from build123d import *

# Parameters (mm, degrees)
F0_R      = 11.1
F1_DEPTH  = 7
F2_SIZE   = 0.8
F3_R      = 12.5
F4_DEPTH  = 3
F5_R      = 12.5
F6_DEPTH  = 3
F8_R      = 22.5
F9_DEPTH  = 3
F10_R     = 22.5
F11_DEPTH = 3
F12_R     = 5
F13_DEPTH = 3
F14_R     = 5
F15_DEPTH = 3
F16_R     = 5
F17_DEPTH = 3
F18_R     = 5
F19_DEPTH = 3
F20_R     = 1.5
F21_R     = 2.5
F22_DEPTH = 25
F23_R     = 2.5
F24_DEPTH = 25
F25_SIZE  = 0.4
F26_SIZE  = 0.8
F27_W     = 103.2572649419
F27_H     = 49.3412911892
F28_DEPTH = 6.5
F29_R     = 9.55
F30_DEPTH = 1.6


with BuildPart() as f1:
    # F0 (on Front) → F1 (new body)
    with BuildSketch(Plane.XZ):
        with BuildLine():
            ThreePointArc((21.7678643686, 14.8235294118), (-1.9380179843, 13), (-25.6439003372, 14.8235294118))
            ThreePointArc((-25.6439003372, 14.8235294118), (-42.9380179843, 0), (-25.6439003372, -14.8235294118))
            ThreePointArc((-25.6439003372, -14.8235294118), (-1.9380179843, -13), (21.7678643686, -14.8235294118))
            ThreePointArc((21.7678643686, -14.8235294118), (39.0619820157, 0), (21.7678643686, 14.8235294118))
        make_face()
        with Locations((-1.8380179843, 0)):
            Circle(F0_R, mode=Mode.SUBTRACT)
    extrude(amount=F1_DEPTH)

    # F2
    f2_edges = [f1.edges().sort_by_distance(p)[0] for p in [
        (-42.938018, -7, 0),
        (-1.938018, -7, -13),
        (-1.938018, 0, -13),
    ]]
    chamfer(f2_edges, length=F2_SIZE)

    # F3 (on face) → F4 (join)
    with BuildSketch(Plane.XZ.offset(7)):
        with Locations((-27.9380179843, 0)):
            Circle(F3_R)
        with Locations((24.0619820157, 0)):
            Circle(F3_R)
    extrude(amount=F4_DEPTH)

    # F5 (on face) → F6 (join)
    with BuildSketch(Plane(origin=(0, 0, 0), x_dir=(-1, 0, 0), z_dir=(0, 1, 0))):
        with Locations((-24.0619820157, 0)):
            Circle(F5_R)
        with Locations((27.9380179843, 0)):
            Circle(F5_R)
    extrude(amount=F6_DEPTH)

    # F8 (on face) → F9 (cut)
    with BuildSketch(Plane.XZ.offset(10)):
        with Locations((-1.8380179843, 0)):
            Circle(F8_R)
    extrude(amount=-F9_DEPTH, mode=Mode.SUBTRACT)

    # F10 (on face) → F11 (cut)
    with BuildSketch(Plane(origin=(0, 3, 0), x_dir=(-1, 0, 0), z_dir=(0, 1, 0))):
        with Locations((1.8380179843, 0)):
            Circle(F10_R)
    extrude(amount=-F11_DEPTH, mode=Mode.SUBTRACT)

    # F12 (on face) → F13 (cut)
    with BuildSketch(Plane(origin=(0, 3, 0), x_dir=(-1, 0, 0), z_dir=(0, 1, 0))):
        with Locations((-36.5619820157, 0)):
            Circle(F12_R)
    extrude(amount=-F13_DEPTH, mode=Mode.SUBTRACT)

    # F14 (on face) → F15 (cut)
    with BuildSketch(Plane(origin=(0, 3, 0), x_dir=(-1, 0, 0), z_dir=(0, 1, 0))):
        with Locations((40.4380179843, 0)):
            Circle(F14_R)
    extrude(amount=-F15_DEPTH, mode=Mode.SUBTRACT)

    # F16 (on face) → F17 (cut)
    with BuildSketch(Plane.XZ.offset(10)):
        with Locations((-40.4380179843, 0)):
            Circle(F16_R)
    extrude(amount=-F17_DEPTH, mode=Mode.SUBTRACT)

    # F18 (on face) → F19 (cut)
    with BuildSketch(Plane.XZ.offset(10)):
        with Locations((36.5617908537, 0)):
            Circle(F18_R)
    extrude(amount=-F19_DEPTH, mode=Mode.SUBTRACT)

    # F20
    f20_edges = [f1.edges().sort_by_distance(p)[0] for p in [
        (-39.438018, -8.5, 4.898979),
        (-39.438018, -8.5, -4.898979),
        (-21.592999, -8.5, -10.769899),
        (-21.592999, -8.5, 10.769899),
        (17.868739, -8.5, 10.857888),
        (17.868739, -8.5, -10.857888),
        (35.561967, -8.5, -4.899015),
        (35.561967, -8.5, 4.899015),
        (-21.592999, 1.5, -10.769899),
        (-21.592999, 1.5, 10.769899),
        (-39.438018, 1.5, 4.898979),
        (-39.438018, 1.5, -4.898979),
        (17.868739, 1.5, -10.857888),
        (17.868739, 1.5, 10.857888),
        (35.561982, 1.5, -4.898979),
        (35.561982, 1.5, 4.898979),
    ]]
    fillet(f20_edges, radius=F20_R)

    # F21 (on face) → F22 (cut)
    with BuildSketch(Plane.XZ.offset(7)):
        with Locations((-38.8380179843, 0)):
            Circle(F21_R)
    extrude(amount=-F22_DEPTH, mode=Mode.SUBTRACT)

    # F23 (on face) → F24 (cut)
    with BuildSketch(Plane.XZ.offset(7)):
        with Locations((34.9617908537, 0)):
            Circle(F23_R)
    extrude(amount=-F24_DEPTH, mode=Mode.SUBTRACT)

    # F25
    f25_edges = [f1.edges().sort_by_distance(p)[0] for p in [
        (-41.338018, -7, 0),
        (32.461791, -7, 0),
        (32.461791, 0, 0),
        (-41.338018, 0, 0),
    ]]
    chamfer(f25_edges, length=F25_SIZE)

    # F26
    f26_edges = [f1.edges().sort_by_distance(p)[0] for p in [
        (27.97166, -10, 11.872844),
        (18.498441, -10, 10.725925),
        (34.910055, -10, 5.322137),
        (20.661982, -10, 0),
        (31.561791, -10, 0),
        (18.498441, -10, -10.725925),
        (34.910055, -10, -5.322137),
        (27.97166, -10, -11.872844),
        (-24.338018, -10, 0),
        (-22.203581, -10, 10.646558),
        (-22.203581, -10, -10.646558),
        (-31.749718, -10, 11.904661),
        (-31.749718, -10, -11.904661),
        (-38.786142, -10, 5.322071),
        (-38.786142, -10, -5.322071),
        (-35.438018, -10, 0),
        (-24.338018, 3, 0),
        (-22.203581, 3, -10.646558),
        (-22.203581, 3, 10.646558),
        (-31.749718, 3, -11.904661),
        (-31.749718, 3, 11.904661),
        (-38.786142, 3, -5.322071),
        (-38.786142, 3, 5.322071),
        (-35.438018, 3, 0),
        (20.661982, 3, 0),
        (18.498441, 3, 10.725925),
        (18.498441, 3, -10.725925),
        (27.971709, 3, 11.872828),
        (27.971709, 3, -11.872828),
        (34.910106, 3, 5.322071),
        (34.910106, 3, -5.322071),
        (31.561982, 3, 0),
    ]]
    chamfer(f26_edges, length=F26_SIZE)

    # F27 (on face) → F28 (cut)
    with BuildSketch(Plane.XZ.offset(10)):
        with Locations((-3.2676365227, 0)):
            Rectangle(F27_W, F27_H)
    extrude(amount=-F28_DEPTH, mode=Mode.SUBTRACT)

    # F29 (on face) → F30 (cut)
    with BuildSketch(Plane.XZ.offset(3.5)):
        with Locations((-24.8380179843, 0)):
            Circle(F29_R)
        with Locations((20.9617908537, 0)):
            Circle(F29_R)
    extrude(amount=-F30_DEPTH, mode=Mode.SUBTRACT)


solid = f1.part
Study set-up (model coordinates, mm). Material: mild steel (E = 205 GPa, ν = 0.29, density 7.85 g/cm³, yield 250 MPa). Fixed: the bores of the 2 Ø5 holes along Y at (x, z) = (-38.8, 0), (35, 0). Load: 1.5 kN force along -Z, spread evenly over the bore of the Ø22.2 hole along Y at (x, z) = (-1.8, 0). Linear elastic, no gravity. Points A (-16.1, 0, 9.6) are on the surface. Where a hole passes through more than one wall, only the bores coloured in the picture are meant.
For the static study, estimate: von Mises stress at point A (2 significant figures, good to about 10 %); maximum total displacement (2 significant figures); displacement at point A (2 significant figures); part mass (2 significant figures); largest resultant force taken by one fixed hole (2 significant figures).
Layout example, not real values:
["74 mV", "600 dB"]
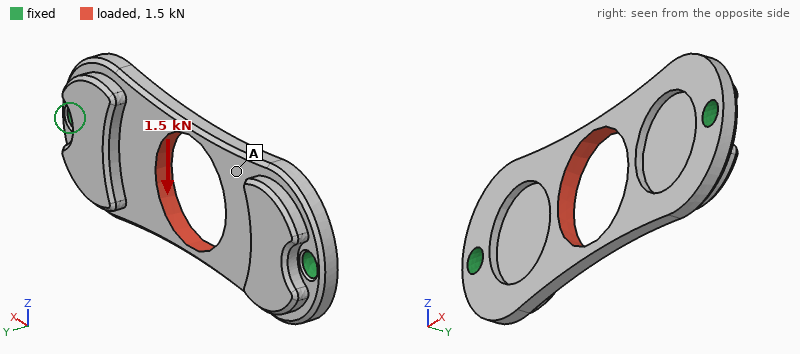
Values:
["19 MPa", "25 µm", "14 µm", "54 g", "750 N"]
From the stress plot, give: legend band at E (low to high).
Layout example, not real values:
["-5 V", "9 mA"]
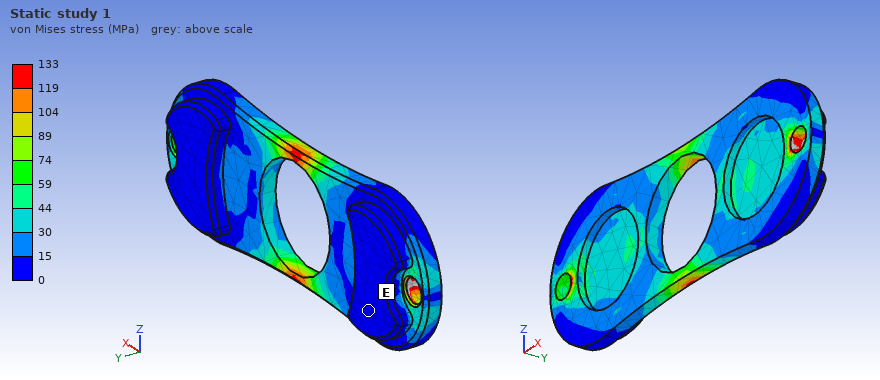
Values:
["0 to 15 MPa"]
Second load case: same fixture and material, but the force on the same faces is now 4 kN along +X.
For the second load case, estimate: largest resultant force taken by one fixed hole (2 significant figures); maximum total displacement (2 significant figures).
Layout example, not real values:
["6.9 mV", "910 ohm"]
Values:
["2.0 kN", "7.3 µm"]
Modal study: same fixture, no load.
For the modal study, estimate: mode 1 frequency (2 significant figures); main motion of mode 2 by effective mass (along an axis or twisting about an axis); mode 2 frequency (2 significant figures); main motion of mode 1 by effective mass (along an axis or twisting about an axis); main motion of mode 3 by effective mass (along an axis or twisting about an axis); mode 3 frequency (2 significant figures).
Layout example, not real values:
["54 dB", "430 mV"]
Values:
["4100 Hz", "twisting about X", "6200 Hz", "along Y", "twisting about Z", "7400 Hz"]
